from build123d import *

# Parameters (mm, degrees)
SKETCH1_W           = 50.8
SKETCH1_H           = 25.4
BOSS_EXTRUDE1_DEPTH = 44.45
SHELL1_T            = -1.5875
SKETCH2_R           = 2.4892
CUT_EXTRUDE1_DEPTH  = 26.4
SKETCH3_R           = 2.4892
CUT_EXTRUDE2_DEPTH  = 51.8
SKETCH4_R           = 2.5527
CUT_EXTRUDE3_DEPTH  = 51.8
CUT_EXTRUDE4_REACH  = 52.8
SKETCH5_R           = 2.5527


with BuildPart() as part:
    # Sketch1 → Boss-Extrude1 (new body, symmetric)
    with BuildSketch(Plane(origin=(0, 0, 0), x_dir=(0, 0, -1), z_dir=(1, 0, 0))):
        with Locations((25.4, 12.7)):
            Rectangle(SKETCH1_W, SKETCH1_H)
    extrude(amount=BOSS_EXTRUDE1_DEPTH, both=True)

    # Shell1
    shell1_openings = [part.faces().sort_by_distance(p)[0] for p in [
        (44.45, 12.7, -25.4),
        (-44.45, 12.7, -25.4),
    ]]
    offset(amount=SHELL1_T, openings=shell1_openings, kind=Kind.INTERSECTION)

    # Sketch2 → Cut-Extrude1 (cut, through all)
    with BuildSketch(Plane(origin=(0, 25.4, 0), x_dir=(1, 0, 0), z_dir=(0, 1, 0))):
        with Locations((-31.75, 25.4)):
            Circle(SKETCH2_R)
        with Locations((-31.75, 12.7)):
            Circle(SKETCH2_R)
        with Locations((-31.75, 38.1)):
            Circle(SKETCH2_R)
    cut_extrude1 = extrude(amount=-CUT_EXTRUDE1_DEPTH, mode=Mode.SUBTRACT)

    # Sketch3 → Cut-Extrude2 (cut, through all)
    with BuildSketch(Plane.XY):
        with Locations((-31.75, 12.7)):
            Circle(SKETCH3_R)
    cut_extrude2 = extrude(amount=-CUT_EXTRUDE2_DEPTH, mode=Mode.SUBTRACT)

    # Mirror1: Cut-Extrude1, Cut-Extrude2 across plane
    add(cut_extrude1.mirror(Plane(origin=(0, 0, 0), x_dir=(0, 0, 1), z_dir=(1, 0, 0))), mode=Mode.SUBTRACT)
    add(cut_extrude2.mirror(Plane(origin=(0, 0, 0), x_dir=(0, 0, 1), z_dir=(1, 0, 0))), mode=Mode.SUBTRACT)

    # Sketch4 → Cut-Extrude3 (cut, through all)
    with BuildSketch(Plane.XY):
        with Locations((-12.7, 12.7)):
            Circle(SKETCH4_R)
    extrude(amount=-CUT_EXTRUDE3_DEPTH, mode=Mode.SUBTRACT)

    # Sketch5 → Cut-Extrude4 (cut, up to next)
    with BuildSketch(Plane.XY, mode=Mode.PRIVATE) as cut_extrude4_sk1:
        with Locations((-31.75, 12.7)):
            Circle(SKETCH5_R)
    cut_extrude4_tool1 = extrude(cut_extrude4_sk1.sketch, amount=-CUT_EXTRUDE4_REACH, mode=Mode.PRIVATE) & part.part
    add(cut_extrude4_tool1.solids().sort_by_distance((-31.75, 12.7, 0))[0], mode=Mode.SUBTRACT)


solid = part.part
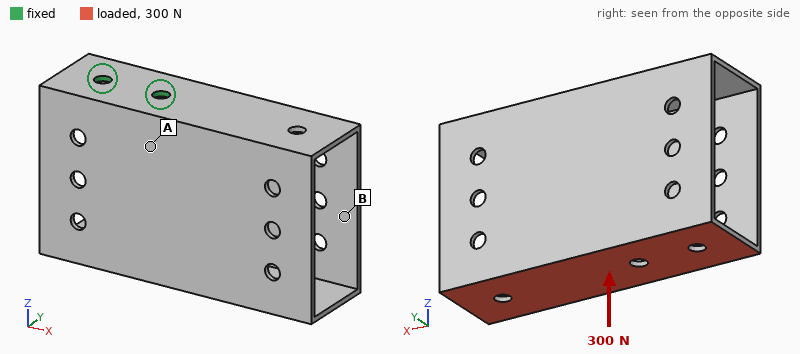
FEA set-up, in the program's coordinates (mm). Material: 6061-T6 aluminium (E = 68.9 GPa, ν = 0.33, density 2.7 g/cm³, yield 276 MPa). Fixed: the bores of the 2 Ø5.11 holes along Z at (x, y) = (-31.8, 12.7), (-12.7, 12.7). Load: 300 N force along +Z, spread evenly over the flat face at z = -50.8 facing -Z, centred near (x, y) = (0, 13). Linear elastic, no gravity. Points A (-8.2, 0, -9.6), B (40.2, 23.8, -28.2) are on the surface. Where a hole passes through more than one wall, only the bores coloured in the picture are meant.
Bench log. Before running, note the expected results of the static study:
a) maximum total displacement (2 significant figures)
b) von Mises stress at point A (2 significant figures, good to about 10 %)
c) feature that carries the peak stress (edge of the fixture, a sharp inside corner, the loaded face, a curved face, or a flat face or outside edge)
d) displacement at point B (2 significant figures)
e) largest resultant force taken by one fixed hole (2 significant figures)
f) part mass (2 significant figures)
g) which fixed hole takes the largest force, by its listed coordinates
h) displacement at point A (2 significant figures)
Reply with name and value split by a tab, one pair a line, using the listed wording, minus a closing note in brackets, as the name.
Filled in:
maximum total displacement	0.39 mm
von Mises stress at point A	20 MPa
feature that carries the peak stress	a flat face or outside edge
displacement at point B	0.32 mm
largest resultant force taken by one fixed hole	410 N
part mass	54 g
which fixed hole takes the largest force, by its listed coordinates	(-12.7, 12.7)
displacement at point A	0.11 mm
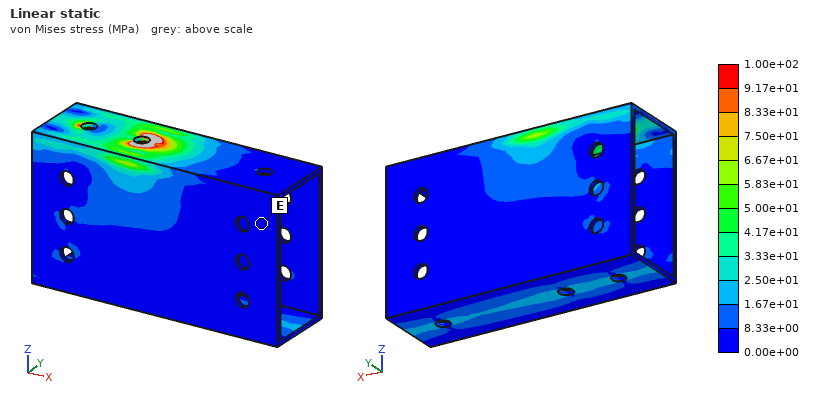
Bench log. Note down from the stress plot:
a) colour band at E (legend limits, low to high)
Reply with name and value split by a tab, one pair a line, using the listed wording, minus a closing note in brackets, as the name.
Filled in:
colour band at E	0.00e+00 to 8.33e+00 MPa
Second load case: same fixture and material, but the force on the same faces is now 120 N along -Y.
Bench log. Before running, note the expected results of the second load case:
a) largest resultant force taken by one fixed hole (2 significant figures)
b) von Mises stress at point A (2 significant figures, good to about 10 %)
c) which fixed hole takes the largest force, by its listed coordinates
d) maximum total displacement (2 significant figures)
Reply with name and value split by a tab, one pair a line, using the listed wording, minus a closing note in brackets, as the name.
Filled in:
largest resultant force taken by one fixed hole	170 N
von Mises stress at point A	23 MPa
which fixed hole takes the largest force, by its listed coordinates	(-12.7, 12.7)
maximum total displacement	1.2 mm
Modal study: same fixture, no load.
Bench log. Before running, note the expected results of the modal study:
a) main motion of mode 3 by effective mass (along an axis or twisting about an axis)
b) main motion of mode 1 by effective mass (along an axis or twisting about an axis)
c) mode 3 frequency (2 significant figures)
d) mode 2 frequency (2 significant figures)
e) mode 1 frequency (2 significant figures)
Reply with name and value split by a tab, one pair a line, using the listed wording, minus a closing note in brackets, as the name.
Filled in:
main motion of mode 3 by effective mass	twisting about Z
main motion of mode 1 by effective mass	along Y
mode 3 frequency	1200 Hz
mode 2 frequency	580 Hz
mode 1 frequency	360 Hz
